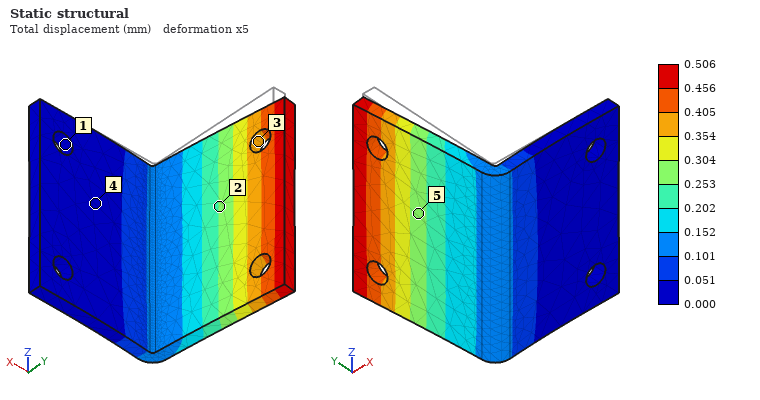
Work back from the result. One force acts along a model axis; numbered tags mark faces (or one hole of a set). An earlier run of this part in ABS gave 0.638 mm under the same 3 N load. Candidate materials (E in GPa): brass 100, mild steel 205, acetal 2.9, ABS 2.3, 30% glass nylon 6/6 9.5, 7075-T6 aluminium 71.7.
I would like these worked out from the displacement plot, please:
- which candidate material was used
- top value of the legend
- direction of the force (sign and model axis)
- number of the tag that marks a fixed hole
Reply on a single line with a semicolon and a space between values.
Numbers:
acetal; 0.506 mm; -X; 1
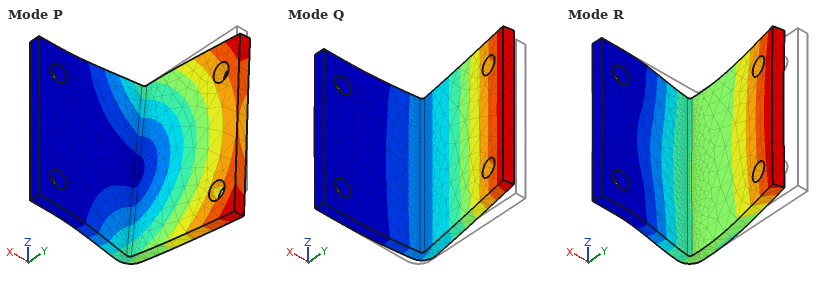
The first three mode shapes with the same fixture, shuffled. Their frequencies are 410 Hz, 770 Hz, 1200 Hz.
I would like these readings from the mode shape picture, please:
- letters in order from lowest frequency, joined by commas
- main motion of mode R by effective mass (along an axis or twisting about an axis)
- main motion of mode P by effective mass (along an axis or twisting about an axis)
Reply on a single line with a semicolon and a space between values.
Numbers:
Q, P, R; along Y; along Z
